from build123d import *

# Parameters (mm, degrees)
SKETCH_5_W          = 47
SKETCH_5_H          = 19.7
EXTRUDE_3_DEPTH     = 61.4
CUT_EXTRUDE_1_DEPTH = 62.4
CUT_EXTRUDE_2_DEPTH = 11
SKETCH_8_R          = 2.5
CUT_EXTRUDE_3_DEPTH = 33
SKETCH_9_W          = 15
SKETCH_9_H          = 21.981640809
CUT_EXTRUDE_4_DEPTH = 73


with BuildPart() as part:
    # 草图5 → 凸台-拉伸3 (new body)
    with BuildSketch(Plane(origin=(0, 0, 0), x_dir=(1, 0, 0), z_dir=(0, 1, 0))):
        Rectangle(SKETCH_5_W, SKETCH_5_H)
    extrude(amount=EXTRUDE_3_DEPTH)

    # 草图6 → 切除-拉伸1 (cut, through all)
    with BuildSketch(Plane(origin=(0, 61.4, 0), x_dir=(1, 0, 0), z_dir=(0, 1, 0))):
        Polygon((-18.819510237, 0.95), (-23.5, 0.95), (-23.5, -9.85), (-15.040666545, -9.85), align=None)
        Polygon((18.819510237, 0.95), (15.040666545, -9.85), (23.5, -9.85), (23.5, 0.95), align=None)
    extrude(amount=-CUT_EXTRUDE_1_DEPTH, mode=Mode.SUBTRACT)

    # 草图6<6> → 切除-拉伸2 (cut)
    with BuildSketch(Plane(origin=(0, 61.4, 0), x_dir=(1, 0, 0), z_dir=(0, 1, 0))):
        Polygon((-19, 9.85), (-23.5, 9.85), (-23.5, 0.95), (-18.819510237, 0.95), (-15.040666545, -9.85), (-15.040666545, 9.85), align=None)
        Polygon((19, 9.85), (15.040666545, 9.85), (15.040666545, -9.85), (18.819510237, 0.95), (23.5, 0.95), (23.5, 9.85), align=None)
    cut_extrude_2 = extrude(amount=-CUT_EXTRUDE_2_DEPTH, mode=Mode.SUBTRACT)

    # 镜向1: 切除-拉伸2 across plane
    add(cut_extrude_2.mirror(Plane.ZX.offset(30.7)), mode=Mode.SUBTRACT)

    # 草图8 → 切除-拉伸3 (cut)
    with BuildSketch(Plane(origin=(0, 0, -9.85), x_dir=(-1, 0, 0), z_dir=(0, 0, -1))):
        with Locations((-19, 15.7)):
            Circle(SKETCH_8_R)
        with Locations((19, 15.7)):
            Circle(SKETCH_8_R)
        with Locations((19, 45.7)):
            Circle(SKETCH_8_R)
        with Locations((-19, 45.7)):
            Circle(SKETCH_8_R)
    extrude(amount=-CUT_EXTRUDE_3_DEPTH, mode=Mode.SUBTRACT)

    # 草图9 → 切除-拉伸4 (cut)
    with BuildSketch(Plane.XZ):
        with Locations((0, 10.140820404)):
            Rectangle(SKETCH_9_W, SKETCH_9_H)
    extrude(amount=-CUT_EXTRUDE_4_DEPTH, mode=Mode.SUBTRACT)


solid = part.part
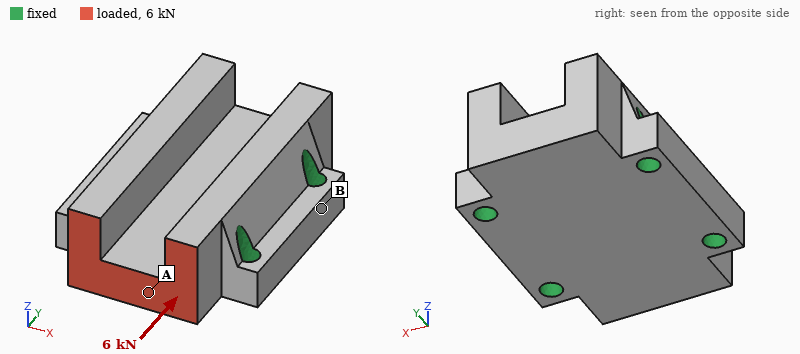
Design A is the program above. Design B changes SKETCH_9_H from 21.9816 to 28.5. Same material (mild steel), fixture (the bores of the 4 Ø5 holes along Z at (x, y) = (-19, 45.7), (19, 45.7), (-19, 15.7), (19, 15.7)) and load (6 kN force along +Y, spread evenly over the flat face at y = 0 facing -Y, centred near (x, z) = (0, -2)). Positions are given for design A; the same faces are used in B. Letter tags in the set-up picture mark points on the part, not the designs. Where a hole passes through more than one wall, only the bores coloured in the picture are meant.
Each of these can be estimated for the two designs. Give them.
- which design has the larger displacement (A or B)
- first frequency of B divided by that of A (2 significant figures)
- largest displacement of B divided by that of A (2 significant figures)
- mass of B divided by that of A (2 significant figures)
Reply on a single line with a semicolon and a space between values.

B; 1.0; 1.3; 0.91
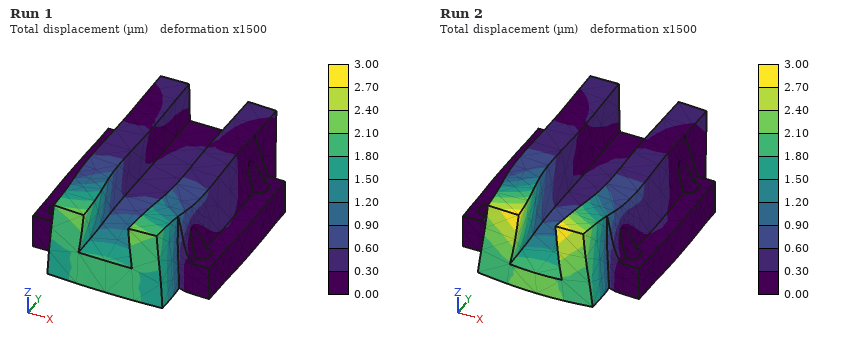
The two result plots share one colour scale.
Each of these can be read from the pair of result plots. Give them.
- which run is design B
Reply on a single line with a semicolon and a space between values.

Run 2
